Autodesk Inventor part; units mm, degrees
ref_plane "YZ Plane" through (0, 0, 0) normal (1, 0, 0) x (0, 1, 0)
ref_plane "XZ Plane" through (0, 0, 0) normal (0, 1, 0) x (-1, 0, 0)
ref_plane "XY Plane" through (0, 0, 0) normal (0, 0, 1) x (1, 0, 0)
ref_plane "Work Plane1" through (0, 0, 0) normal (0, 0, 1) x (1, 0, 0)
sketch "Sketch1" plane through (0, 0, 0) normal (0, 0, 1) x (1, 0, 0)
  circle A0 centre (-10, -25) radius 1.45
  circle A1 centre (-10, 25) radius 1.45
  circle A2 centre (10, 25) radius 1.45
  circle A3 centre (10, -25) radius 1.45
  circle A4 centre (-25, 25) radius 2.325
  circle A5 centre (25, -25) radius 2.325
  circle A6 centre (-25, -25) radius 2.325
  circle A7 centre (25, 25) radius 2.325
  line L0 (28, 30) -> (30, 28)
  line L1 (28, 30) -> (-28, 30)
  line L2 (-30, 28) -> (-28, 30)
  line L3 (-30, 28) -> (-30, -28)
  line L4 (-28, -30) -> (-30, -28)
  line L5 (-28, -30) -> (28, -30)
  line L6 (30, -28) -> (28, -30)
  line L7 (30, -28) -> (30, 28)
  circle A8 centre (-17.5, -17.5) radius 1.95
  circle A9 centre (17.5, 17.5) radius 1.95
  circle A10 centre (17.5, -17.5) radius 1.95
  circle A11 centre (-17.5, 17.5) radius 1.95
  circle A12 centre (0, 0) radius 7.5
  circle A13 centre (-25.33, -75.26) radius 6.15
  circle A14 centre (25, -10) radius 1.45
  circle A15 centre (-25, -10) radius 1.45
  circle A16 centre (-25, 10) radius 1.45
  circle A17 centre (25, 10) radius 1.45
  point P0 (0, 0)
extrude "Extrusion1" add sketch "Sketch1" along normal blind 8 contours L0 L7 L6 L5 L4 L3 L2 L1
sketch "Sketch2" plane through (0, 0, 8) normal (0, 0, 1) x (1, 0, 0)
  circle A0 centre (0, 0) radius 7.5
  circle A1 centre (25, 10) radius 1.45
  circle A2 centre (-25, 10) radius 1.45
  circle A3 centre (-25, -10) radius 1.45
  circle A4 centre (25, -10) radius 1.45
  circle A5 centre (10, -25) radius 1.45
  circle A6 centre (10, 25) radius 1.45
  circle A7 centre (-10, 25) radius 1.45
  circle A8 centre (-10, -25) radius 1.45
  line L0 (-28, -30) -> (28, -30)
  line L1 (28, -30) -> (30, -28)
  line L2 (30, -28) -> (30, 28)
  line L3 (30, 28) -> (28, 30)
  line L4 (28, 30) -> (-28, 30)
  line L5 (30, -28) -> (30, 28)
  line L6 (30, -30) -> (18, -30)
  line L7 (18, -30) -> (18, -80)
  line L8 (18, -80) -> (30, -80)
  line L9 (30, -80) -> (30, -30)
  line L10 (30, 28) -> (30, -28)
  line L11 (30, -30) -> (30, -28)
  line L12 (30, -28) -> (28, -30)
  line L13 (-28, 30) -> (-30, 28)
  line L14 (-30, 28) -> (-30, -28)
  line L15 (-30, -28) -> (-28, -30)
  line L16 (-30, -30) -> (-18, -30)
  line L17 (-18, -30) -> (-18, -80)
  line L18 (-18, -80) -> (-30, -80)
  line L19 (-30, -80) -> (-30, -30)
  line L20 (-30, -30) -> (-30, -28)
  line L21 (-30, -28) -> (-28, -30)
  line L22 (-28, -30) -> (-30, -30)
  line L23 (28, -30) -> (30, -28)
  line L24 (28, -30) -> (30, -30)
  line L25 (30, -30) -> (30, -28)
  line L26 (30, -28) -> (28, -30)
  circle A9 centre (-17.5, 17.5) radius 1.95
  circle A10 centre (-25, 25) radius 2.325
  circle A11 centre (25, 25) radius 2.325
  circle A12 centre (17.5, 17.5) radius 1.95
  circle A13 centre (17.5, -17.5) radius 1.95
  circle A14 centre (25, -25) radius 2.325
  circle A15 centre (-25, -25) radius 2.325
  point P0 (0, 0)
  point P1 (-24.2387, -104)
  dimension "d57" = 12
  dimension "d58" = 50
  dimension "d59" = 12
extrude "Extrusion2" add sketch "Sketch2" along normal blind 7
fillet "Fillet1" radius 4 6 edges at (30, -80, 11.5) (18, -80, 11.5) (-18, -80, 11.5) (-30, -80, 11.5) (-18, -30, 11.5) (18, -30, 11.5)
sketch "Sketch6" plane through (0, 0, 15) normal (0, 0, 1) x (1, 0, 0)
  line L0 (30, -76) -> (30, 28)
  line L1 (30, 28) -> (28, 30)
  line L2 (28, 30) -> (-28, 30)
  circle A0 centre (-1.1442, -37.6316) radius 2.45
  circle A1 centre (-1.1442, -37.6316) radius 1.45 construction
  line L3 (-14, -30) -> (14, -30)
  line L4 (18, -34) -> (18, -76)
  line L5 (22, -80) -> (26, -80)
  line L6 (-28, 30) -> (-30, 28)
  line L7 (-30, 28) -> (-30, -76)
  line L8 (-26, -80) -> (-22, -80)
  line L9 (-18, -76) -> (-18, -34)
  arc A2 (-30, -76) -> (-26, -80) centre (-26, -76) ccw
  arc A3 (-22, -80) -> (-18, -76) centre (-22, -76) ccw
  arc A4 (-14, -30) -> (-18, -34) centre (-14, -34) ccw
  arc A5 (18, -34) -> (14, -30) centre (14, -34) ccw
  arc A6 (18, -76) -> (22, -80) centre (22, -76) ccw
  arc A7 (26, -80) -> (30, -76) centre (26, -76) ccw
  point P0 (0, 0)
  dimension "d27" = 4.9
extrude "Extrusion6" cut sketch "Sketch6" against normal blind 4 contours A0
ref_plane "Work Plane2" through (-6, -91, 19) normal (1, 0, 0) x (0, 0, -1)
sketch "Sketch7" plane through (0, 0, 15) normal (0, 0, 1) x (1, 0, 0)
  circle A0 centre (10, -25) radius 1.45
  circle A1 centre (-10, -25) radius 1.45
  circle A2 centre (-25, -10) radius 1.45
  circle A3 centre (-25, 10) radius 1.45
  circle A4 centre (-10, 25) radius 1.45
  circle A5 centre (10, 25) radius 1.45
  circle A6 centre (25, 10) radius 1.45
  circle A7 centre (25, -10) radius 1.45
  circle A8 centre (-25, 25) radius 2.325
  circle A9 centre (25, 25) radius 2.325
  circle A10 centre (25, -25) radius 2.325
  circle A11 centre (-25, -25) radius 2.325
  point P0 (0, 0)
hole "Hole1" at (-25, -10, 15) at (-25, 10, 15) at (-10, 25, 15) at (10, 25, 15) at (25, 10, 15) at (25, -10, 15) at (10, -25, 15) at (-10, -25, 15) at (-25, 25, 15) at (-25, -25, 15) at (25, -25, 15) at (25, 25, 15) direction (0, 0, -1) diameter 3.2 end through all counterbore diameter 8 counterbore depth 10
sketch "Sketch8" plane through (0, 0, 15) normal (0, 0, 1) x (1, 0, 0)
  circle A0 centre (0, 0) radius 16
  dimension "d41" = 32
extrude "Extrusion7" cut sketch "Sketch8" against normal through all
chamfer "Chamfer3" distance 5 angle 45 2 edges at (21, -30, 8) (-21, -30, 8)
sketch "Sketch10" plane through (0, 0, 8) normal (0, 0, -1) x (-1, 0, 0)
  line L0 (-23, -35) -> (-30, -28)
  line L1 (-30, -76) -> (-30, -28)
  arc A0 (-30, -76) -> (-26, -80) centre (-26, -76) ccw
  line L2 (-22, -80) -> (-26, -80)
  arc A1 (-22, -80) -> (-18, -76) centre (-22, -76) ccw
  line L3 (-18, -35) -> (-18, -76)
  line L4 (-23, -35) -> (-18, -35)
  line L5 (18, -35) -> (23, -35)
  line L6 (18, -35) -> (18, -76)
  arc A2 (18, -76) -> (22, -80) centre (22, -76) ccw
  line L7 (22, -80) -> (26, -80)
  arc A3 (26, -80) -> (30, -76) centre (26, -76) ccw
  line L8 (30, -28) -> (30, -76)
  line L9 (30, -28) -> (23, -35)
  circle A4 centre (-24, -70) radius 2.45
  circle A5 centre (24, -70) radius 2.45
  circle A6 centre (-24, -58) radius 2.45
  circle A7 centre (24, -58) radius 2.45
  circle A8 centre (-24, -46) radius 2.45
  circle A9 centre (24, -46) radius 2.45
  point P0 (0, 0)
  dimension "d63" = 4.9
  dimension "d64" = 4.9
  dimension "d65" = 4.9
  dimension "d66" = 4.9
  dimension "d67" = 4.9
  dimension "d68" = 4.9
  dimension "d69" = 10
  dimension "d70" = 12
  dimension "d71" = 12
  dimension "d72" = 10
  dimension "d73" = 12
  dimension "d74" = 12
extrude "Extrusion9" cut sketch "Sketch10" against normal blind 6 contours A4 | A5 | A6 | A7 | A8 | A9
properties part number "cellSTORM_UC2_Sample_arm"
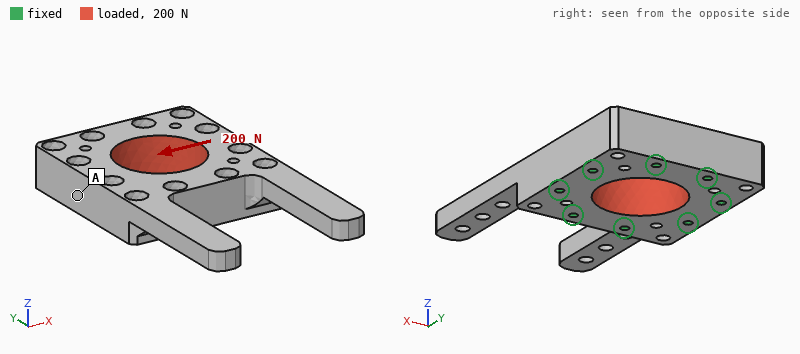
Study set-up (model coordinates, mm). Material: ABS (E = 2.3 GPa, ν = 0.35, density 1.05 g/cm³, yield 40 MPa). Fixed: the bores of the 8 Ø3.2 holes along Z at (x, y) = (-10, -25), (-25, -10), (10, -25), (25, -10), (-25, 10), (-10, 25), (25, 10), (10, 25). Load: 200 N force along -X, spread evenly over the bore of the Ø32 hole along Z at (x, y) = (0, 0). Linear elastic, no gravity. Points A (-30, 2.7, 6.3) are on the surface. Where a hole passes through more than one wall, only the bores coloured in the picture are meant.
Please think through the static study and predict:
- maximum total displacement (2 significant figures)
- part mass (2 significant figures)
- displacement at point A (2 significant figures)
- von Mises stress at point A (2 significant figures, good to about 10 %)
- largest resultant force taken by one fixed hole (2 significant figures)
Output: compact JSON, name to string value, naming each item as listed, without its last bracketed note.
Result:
{"maximum total displacement": "7.0 µm", "part mass": "45 g", "displacement at point A": "2.5 µm", "von Mises stress at point A": "0.15 MPa", "largest resultant force taken by one fixed hole": "29 N"}
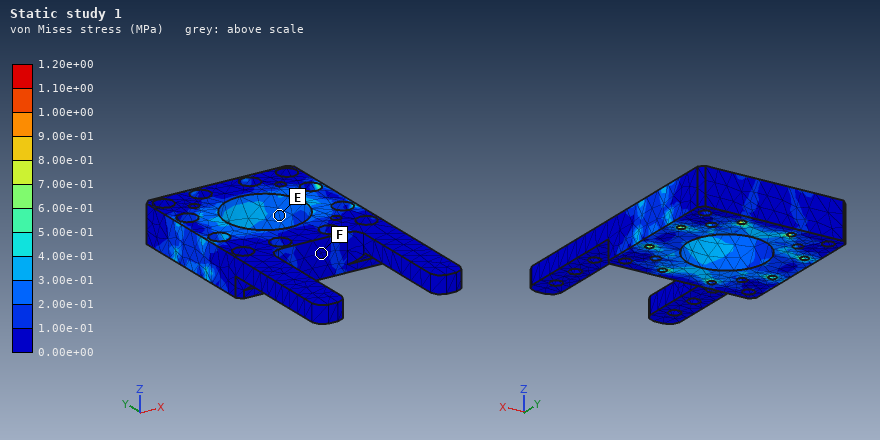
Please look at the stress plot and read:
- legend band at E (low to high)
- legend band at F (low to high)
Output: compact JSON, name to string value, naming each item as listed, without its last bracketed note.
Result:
{"legend band at E": "2.00e-01 to 3.00e-01 MPa", "legend band at F": "0.00e+00 to 1.00e-01 MPa"}
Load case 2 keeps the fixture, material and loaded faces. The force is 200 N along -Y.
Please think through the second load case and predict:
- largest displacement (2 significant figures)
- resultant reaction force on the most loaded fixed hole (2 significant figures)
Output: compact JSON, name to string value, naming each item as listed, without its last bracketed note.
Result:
{"largest displacement": "11 µm", "resultant reaction force on the most loaded fixed hole": "29 N"}
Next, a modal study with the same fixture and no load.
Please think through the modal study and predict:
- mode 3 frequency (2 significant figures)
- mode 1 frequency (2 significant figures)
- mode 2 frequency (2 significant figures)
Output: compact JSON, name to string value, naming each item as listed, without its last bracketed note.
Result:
{"mode 3 frequency": "920 Hz", "mode 1 frequency": "610 Hz", "mode 2 frequency": "610 Hz"}
